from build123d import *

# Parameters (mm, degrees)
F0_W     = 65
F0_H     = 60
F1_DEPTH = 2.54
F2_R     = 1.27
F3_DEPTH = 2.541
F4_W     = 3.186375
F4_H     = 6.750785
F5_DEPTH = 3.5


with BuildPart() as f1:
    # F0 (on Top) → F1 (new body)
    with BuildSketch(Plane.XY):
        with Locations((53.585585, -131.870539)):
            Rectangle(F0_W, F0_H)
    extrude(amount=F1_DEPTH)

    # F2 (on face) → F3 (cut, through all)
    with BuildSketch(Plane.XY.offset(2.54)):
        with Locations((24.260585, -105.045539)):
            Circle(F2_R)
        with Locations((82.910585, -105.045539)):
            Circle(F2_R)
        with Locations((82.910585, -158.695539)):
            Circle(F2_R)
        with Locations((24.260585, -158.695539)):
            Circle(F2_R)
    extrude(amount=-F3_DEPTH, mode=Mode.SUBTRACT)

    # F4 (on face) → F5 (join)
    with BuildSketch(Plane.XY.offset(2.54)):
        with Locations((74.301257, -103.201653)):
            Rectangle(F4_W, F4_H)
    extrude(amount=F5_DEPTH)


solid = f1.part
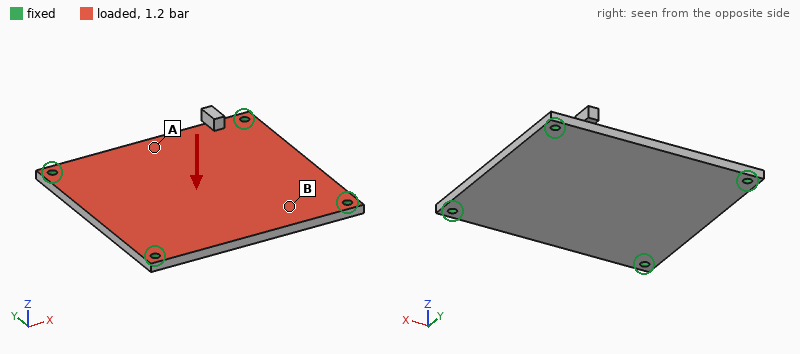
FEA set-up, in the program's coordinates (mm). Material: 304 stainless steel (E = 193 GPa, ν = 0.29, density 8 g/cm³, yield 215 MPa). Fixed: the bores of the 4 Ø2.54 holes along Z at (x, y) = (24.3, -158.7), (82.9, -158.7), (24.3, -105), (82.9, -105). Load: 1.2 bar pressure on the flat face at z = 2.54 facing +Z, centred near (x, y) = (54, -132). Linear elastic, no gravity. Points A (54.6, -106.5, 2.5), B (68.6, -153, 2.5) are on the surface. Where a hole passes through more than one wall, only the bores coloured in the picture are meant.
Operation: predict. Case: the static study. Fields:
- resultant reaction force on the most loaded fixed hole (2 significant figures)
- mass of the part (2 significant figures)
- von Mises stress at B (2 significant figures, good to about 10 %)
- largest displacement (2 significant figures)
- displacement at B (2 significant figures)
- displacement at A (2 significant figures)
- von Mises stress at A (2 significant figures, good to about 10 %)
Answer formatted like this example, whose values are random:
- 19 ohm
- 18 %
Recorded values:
- 120 N
- 79 g
- 11 MPa
- 37 µm
- 18 µm
- 24 µm
- 23 MPa
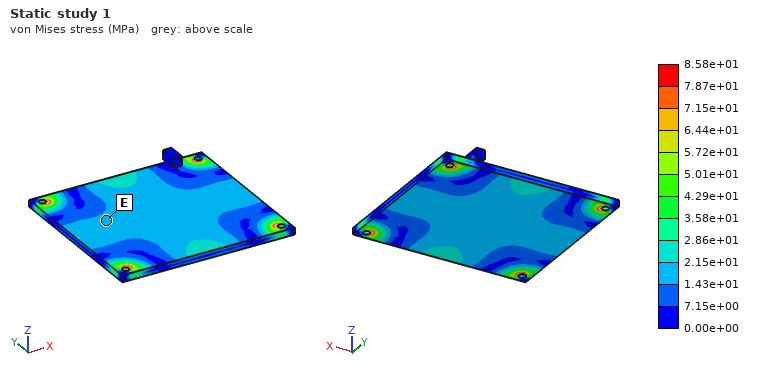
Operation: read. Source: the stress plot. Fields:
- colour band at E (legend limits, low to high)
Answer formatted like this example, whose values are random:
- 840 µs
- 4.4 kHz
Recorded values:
- 1.43e+01 to 2.15e+01 MPa
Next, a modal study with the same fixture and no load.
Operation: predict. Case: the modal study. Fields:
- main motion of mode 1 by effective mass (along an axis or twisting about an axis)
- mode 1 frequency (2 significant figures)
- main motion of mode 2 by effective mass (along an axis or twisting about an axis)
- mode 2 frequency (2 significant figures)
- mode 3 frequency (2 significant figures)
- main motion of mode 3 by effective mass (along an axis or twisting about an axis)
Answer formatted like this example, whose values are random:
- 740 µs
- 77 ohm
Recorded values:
- along Z
- 2400 Hz
- twisting about X
- 4200 Hz
- 4600 Hz
- twisting about Y
